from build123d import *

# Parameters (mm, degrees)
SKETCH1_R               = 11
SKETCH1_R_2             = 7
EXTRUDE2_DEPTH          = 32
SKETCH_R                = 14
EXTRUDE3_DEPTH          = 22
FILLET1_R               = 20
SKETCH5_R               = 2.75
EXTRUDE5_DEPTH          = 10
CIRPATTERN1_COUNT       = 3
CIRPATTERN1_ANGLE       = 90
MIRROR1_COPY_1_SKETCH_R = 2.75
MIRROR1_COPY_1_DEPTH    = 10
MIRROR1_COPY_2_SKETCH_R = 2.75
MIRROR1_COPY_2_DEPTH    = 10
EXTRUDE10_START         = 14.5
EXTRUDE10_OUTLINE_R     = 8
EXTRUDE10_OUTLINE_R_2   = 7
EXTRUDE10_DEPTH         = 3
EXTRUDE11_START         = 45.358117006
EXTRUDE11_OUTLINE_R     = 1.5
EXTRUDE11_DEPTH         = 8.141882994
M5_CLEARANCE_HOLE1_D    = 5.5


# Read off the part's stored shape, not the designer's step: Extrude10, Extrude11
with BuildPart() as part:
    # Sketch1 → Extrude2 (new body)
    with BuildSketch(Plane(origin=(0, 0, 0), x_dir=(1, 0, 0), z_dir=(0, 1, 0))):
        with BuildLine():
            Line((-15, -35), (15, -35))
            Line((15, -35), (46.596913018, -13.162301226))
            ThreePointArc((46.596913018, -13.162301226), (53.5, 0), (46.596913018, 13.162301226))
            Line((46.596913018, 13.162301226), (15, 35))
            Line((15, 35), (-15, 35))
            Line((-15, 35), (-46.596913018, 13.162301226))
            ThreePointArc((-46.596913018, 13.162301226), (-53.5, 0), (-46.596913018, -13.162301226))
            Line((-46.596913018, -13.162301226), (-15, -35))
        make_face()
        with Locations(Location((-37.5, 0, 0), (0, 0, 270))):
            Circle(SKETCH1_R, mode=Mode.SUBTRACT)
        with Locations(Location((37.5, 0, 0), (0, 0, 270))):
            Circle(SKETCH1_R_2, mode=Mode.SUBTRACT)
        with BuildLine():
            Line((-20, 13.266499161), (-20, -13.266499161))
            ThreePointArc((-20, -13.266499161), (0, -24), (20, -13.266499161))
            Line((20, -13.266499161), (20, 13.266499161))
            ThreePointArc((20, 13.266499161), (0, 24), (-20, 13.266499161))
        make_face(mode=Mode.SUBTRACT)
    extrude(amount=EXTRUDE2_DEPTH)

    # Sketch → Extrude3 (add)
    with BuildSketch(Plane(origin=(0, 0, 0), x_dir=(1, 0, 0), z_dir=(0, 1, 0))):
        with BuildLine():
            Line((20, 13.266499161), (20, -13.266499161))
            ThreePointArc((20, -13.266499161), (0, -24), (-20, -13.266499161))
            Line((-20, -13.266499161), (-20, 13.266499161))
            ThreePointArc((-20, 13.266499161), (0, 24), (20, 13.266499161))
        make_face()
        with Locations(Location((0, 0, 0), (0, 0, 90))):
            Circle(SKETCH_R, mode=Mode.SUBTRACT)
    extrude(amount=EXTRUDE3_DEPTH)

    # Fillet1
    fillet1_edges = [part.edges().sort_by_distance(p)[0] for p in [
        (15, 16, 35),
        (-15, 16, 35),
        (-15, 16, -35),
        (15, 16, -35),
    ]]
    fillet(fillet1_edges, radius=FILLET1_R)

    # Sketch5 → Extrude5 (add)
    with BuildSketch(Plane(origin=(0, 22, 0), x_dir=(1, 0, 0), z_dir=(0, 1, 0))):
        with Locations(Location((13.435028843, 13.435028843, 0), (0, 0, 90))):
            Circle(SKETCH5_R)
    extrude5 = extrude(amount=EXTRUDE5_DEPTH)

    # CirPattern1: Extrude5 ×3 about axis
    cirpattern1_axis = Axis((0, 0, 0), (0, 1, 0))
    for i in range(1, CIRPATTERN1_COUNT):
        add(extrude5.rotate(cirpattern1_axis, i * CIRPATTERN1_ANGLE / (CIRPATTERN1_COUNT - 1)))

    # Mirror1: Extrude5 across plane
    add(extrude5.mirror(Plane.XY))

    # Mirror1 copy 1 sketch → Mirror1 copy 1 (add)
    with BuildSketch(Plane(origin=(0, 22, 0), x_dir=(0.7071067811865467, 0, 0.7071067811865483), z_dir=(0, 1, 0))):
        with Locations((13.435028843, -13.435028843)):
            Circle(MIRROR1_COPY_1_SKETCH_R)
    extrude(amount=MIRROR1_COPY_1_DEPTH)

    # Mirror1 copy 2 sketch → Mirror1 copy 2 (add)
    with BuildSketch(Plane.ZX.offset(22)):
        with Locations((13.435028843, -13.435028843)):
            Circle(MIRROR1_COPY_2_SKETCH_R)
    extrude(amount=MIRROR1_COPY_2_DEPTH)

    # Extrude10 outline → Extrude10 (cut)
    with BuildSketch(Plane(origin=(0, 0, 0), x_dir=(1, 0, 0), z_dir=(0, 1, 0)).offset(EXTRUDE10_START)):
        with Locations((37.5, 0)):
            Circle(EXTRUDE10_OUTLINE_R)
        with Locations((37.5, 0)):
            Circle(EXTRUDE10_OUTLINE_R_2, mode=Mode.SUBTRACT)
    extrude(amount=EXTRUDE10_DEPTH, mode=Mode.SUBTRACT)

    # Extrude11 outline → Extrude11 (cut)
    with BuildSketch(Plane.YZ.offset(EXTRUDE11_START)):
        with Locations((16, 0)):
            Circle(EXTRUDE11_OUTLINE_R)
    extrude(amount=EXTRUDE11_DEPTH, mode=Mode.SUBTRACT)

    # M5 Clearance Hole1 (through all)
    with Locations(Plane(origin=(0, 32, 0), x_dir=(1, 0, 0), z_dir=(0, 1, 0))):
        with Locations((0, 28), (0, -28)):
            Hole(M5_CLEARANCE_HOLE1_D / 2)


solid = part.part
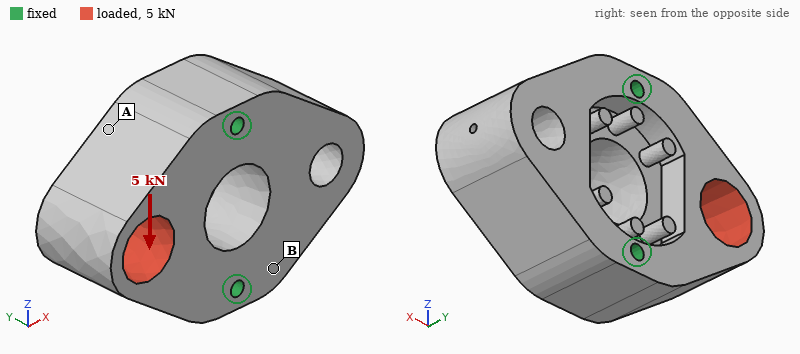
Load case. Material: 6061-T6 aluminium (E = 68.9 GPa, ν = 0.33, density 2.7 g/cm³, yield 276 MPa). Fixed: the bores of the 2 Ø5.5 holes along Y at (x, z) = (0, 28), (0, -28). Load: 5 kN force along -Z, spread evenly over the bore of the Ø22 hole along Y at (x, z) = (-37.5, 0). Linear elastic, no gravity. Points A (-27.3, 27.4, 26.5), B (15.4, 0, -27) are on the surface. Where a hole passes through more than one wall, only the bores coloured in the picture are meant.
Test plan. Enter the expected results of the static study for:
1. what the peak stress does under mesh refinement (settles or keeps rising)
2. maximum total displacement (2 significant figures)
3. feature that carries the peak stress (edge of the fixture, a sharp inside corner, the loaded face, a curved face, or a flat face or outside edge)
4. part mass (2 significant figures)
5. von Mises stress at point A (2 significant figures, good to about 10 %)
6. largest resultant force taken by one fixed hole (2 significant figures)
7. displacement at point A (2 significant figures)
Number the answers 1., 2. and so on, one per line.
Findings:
1. keeps rising
2. 20 µm
3. edge of the fixture
4. 340 g
5. 7.0 MPa
6. 3.9 kN
7. 7.9 µm
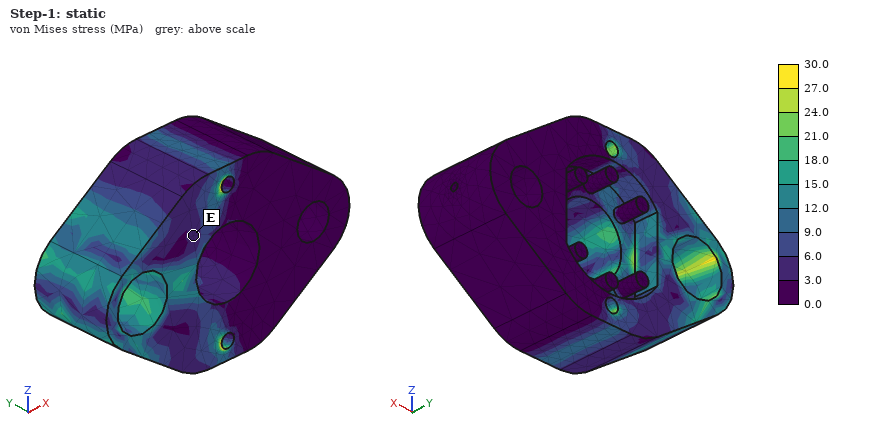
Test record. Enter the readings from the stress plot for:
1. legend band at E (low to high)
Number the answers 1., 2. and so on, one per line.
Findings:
1. 3.0 to 6.0 MPa
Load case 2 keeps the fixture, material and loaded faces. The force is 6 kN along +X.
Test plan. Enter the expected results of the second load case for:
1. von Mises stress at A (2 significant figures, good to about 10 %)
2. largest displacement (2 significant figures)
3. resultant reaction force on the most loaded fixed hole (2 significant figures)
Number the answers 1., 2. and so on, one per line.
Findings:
1. 4.8 MPa
2. 7.7 µm
3. 3.2 kN
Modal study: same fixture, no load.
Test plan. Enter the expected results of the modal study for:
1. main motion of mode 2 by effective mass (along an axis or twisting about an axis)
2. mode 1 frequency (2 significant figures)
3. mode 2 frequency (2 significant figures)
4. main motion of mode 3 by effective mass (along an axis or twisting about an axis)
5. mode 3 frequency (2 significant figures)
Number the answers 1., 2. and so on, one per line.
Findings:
1. along Y
2. 7100 Hz
3. 8400 Hz
4. twisting about Y
5. 12 kHz
